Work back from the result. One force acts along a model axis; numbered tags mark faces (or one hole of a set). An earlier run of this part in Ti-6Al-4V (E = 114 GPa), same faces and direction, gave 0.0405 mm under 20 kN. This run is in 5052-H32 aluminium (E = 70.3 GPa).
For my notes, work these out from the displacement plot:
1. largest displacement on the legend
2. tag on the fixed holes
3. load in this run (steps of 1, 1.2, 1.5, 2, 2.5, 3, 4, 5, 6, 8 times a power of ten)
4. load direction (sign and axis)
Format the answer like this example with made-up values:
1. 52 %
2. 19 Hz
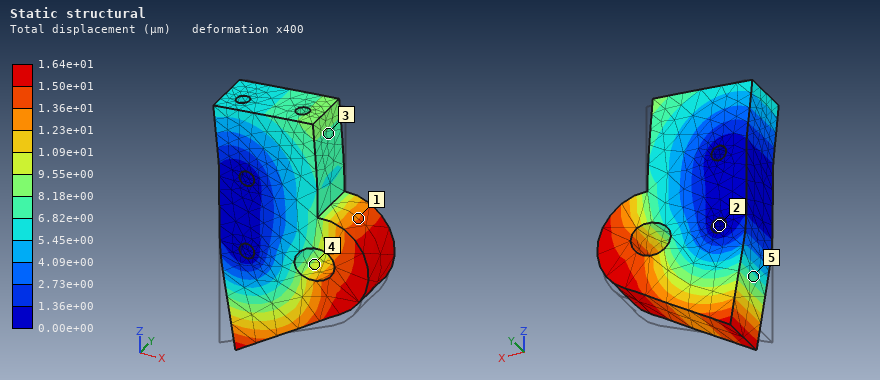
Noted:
1. 1.64e+01 µm
2. 2
3. 5 kN
4. +Z
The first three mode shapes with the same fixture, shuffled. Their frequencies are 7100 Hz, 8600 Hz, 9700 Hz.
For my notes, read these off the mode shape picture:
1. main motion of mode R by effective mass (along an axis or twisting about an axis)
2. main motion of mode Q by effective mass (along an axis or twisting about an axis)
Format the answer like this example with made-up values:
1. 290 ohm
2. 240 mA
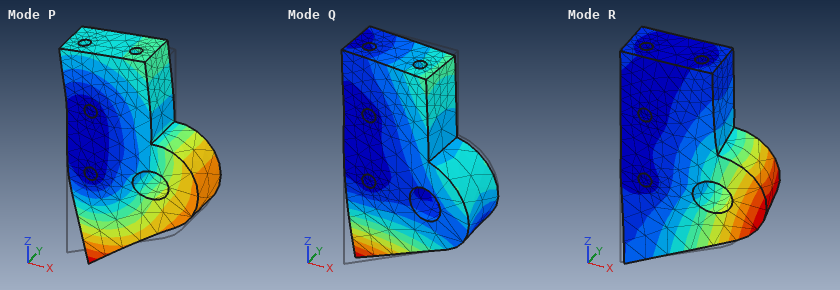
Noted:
1. along Y
2. twisting about X
